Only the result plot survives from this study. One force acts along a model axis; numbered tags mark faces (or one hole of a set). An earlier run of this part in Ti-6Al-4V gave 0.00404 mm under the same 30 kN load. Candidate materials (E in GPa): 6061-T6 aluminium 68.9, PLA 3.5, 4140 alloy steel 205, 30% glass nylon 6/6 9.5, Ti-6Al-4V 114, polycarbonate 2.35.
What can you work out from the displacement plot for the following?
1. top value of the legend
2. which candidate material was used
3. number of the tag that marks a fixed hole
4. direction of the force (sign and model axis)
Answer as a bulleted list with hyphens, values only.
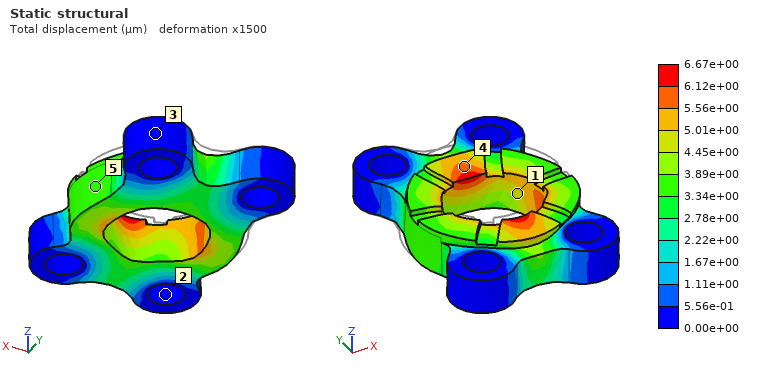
- 6.67e+00 µm
- 6061-T6 aluminium
- 2
- -Y
